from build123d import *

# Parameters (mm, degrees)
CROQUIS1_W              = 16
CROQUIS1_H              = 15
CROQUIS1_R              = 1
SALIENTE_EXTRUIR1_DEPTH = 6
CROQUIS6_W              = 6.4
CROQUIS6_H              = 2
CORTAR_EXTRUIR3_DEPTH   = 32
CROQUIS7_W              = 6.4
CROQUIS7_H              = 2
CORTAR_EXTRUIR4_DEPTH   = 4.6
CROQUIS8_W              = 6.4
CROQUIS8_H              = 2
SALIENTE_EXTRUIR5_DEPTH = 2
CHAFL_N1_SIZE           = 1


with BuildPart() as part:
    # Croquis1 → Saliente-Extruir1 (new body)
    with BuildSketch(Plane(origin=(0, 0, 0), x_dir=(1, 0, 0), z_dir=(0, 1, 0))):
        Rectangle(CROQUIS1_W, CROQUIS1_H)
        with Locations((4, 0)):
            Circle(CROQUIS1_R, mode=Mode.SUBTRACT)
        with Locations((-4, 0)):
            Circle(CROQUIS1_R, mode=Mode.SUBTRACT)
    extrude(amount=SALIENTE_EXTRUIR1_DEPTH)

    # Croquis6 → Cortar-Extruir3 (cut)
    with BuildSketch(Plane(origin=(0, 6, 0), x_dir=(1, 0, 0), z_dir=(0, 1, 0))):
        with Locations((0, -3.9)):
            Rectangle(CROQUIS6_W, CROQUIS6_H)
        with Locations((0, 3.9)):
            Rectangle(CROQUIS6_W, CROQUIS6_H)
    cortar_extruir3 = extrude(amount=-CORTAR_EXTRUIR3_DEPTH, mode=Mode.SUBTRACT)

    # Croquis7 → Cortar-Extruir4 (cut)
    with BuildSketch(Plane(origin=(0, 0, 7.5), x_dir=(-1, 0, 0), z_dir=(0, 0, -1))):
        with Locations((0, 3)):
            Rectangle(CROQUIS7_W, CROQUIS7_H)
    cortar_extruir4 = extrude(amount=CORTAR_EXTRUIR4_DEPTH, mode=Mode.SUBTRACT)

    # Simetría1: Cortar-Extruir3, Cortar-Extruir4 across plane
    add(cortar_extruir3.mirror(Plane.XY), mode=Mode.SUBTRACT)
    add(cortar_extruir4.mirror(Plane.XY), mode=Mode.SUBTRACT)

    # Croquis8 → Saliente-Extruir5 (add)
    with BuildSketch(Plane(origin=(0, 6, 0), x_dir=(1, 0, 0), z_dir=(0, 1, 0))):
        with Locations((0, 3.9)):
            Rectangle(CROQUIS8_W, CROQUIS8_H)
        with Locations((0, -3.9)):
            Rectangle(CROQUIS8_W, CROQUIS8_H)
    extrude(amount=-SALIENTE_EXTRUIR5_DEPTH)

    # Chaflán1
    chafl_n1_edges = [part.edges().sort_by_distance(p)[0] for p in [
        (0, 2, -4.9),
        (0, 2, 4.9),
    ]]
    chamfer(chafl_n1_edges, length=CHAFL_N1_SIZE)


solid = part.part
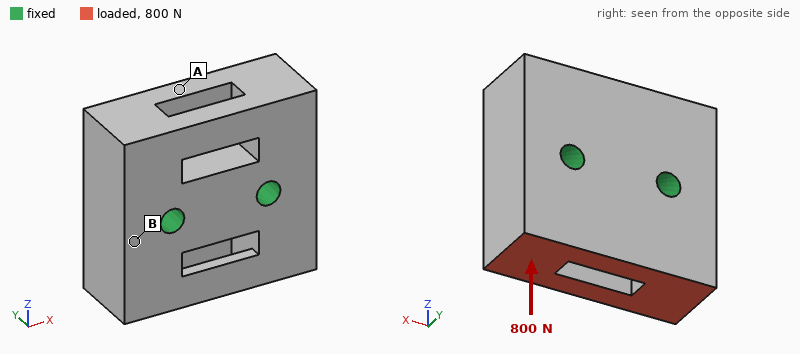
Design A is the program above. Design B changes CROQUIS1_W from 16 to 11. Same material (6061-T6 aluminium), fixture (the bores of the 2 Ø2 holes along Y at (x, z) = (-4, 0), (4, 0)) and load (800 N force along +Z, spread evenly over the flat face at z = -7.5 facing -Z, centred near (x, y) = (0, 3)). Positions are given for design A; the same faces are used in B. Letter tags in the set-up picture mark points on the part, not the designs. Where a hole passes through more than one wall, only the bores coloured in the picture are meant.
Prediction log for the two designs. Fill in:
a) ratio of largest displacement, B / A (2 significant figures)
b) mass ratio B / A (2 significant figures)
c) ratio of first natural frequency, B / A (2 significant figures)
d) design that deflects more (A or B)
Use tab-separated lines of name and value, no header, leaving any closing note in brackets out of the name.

ratio of largest displacement, B / A	1.7
mass ratio B / A	0.63
ratio of first natural frequency, B / A	1.1
design that deflects more	B
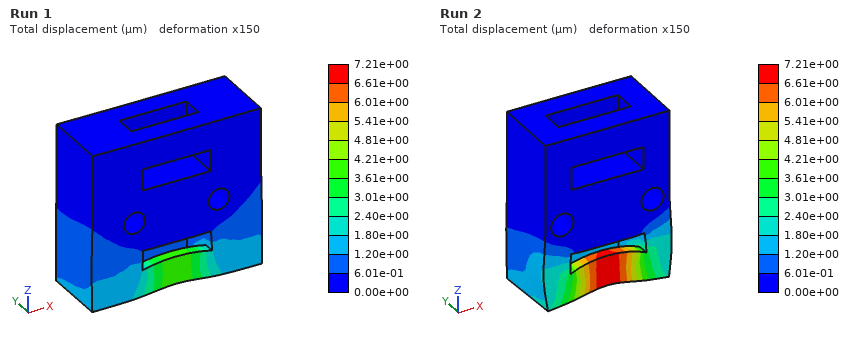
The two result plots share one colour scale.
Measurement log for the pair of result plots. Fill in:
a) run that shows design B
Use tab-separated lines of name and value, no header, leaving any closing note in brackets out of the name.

run that shows design B	Run 2
